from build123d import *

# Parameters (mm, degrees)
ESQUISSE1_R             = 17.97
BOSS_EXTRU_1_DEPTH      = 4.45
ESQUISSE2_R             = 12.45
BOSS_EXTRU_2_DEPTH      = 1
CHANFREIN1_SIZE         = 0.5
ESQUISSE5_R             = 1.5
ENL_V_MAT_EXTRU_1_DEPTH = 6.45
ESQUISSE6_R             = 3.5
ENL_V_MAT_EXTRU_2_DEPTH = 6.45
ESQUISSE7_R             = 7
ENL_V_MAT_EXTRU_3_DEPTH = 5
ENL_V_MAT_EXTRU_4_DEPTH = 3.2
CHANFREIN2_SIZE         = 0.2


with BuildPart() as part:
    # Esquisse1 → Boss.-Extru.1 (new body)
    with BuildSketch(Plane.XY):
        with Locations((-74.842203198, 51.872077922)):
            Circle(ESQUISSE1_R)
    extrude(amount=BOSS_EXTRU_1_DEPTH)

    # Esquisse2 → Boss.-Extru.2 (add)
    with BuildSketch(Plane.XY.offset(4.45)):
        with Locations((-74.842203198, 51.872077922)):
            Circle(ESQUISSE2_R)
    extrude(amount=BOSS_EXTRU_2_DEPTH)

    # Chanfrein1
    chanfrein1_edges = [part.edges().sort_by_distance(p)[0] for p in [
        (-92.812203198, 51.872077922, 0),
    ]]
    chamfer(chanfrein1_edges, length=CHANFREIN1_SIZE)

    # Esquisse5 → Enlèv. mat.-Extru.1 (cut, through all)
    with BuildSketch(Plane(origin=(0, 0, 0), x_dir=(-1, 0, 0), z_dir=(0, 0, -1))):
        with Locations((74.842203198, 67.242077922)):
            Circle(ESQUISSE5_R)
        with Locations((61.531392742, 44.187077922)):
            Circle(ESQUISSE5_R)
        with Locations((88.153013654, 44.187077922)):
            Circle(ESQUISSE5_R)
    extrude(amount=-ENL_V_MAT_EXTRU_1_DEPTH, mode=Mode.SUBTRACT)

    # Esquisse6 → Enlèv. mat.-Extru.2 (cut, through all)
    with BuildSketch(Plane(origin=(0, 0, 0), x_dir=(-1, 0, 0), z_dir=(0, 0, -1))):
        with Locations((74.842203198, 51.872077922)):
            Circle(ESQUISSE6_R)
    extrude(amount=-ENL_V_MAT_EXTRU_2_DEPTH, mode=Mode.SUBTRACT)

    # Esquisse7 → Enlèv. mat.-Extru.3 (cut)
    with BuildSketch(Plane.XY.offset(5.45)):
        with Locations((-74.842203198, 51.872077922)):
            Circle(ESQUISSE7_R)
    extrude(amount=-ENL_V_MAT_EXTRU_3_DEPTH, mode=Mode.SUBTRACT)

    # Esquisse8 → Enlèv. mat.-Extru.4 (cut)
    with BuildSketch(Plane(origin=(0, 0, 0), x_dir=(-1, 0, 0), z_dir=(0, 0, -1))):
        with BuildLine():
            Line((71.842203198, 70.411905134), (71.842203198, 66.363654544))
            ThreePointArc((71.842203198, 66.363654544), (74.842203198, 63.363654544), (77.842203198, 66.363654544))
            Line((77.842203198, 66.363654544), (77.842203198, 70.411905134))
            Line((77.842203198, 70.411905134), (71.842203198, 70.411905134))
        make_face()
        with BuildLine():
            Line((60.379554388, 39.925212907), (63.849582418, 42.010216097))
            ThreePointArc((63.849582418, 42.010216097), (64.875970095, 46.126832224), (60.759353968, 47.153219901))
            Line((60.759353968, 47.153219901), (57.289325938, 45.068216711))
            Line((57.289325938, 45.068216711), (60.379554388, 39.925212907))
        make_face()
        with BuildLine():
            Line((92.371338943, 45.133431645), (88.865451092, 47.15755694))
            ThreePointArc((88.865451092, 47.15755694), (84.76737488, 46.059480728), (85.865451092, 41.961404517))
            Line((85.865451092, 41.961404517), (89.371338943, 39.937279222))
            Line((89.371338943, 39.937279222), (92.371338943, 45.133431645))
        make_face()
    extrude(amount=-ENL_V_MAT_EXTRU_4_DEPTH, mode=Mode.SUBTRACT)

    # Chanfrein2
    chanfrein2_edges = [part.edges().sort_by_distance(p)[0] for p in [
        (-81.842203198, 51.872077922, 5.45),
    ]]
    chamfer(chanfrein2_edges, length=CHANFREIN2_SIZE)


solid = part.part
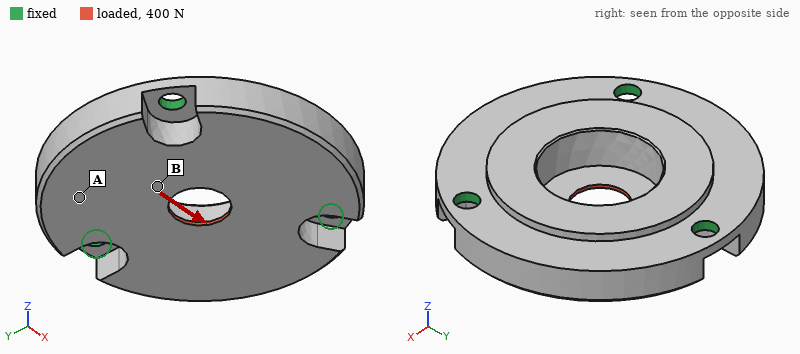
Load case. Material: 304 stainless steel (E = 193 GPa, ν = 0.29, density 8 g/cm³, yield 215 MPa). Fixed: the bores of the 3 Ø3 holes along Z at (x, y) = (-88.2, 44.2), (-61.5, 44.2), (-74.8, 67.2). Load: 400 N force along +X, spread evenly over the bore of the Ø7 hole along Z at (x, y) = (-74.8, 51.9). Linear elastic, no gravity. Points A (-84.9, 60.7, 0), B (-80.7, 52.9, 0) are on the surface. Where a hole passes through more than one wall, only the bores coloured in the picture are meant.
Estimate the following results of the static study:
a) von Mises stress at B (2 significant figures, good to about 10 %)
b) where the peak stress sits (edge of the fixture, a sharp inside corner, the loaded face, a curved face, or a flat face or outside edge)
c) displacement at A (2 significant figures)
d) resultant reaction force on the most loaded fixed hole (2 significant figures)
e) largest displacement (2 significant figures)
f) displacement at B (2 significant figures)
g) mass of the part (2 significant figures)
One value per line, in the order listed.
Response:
34 MPa
the loaded face
1.3 µm
150 N
1.9 µm
1.3 µm
31 g
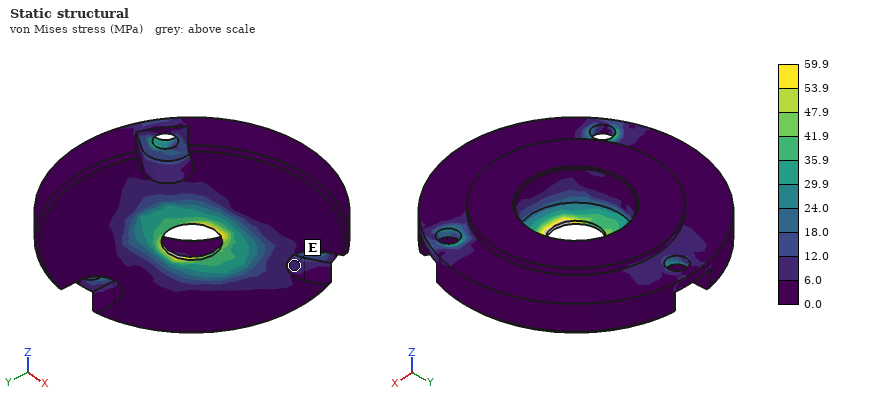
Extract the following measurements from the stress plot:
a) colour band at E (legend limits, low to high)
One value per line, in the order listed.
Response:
6.0 to 12.0 MPa
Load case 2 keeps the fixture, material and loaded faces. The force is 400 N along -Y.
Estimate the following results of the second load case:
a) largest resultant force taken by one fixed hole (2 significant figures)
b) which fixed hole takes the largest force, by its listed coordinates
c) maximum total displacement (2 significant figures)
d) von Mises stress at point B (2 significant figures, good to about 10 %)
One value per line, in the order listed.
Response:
160 N
(-74.8, 67.2)
2.1 µm
22 MPa
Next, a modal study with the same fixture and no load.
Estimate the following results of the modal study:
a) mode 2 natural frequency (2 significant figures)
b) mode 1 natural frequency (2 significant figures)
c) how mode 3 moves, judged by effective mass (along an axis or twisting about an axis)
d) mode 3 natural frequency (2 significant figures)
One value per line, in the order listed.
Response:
13 kHz
13 kHz
along Z
16 kHz
